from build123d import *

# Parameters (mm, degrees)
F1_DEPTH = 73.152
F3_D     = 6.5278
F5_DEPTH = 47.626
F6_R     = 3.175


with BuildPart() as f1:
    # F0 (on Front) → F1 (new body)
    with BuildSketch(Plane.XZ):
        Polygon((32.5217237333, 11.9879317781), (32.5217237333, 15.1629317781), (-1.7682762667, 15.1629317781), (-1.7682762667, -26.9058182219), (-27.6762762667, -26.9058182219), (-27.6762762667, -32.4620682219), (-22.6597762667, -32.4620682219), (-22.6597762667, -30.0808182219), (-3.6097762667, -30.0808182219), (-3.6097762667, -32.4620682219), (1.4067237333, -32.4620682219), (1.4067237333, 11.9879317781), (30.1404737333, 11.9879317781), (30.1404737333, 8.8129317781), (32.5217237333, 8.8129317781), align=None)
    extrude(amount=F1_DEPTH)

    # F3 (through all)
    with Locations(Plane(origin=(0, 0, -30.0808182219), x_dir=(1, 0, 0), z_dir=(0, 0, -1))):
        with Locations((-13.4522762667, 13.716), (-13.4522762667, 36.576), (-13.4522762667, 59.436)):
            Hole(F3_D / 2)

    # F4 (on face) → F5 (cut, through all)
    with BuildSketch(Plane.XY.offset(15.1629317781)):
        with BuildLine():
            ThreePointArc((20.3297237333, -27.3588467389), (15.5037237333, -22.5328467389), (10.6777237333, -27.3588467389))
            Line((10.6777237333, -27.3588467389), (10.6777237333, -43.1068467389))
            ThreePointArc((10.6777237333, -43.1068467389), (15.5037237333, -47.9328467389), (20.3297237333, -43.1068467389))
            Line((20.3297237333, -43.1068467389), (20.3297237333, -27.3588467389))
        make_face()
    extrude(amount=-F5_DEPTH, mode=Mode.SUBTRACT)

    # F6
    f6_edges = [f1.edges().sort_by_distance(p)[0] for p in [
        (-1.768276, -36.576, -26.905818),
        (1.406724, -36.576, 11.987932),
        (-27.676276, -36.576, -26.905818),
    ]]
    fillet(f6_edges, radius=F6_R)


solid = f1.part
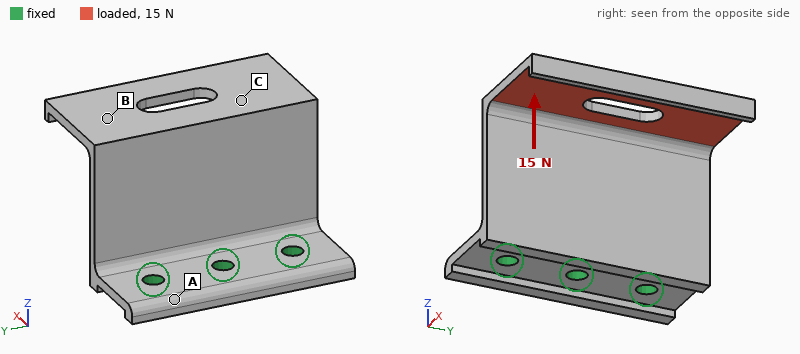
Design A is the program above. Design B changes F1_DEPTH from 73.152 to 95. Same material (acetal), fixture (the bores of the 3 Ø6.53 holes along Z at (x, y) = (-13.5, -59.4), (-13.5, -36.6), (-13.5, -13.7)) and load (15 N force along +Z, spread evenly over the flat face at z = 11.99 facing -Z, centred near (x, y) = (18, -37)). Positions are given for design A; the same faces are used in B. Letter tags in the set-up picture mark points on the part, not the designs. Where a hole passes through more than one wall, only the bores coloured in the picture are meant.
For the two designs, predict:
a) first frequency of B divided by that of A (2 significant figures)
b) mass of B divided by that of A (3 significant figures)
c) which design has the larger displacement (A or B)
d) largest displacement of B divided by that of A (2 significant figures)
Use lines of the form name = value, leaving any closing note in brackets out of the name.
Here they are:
first frequency of B divided by that of A = 0.95
mass of B divided by that of A = 1.31
which design has the larger displacement = A
largest displacement of B divided by that of A = 0.84
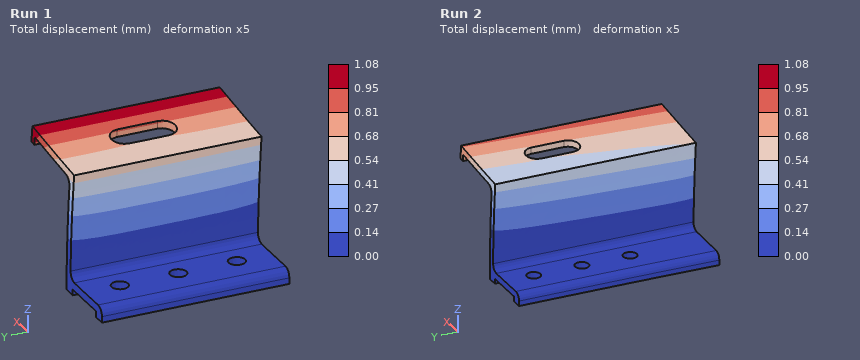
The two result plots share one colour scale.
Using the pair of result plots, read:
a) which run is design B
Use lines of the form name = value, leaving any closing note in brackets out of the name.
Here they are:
which run is design B = Run 2
